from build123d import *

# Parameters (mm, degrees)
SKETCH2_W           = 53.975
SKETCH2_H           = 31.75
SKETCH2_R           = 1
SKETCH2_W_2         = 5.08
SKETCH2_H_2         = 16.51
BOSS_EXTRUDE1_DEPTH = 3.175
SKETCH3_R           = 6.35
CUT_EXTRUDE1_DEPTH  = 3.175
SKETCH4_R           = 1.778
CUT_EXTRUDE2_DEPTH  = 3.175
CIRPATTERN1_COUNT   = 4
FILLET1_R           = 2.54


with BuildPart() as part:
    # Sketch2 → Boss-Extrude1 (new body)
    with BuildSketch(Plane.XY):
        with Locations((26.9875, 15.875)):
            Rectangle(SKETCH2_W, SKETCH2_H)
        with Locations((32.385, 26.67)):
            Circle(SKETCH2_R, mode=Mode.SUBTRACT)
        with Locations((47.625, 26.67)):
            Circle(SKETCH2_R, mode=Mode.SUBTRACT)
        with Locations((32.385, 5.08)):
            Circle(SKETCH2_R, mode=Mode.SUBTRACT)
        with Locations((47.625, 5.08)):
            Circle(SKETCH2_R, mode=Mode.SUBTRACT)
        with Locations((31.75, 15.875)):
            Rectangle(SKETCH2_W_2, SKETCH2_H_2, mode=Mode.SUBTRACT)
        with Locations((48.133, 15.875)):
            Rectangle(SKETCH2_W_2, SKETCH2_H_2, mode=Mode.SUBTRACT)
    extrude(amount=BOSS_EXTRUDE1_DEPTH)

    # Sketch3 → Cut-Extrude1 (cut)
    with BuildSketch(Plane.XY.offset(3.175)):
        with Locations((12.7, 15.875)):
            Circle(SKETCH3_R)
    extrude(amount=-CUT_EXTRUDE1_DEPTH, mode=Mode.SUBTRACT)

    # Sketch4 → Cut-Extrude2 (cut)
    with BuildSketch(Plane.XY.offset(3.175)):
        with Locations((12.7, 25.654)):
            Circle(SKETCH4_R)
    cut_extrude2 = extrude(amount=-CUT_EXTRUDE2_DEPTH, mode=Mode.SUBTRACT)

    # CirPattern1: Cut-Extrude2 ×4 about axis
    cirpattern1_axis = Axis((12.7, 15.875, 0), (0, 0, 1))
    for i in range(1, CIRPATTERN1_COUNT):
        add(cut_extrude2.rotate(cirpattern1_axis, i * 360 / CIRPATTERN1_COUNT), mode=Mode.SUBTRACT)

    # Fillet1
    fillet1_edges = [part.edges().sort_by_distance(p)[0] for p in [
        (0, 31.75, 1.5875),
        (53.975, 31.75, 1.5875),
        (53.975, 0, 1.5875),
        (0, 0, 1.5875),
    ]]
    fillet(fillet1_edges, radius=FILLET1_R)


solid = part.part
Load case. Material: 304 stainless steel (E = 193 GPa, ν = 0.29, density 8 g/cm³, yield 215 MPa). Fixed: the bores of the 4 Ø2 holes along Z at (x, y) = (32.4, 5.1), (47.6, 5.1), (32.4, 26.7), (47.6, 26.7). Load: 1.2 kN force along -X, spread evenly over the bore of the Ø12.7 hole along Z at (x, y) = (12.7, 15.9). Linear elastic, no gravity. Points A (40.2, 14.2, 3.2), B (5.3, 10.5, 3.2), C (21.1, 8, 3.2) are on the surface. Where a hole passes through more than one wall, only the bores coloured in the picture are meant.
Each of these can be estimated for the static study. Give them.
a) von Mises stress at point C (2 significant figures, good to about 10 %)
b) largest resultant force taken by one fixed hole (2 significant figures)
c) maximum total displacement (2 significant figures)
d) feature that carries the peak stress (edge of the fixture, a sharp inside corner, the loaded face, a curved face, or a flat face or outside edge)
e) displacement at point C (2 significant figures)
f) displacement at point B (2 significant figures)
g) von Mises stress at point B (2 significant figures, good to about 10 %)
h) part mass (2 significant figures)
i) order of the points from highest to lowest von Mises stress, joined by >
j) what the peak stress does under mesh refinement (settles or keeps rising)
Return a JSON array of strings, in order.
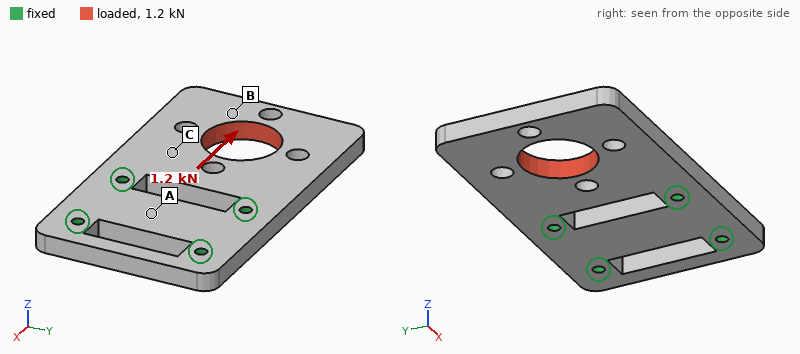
["18 MPa", "560 N", "4.3 µm", "edge of the fixture", "1.5 µm", "3.3 µm", "9.4 MPa", "35 g", "C > B > A", "keeps rising"]
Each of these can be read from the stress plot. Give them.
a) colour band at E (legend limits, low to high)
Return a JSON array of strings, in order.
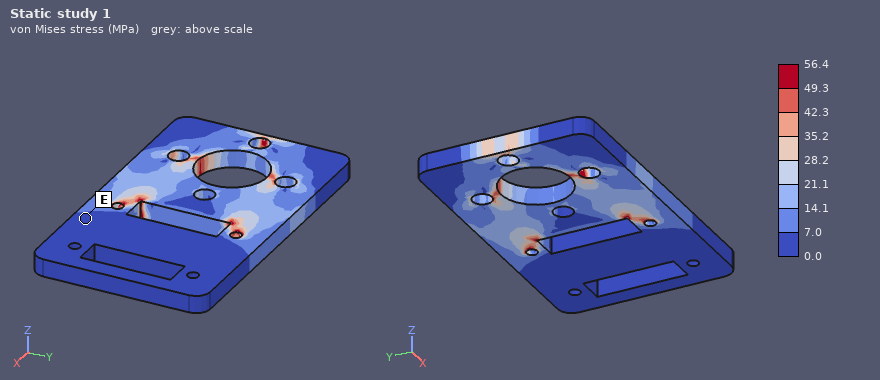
["0.0 to 7.0 MPa"]
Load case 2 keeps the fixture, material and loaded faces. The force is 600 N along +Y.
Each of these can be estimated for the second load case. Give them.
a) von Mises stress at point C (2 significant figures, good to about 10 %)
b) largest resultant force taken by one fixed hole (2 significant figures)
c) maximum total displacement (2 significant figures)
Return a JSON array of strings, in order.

["12 MPa", "500 N", "10 µm"]
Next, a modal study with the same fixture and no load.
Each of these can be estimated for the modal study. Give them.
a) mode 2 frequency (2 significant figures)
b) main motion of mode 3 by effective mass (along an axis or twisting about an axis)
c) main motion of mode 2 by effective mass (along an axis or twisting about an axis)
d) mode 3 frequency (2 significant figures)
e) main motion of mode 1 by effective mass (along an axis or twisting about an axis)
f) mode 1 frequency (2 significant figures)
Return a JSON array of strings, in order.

["5000 Hz", "along Y", "twisting about X", "11 kHz", "along Z", "2000 Hz"]
